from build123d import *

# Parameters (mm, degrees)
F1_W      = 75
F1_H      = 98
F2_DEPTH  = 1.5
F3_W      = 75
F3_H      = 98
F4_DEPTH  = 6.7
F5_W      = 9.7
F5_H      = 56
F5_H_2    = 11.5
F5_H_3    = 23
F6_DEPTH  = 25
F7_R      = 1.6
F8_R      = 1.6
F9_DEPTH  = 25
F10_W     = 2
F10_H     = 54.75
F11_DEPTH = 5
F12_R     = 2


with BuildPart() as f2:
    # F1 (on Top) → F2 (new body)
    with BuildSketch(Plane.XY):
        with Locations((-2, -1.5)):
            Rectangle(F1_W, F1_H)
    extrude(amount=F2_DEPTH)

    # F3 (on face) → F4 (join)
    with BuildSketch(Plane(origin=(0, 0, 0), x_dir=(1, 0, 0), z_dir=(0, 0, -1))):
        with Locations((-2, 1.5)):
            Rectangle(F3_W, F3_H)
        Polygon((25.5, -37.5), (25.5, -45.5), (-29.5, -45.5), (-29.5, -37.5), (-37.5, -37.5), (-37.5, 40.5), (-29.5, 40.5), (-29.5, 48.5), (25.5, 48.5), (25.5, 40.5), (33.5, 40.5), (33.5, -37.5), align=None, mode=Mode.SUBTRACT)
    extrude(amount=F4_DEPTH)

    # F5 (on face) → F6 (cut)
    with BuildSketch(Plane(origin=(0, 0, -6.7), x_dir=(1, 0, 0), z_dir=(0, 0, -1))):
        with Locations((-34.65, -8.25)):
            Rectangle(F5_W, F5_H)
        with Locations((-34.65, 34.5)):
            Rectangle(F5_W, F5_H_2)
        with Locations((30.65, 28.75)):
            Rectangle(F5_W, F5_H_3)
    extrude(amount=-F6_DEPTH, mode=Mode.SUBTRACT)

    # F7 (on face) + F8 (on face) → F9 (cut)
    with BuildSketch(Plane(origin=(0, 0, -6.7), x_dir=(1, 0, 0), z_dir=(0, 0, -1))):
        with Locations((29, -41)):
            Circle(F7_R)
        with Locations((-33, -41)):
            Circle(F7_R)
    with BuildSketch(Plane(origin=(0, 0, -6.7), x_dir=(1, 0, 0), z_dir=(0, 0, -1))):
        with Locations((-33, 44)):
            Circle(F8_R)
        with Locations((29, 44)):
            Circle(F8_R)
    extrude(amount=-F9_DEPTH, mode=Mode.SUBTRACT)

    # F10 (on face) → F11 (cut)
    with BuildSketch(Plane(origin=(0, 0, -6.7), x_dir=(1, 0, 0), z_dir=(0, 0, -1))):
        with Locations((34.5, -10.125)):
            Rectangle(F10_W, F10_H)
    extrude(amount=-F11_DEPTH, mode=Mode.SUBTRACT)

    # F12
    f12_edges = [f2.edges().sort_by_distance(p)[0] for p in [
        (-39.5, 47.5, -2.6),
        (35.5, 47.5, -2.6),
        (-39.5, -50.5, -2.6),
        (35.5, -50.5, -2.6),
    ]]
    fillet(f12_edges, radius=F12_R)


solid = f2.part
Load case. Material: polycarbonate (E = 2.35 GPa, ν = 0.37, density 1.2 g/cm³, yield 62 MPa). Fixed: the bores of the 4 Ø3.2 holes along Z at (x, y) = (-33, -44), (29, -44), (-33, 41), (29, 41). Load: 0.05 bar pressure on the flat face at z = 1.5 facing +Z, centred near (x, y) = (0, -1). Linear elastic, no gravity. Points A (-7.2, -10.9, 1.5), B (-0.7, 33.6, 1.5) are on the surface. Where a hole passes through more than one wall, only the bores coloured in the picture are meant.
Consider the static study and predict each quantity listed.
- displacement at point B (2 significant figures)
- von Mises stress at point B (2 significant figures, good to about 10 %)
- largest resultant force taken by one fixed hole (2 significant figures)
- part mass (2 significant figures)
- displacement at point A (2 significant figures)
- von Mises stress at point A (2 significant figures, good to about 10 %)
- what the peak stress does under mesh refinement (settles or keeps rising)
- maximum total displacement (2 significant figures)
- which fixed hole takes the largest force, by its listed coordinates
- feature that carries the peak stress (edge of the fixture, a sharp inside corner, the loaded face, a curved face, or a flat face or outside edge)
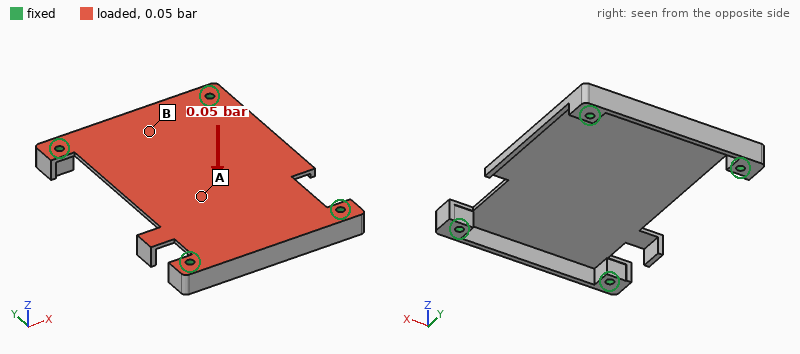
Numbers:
0.36 mm
1.7 MPa
13 N
17 g
1.3 mm
3.8 MPa
keeps rising
1.5 mm
(29, 41)
a sharp inside corner
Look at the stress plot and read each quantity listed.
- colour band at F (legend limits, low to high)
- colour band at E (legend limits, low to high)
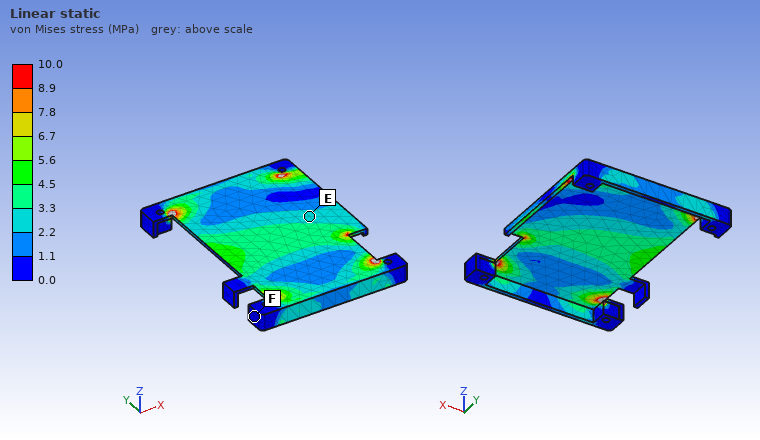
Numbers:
0.0 to 1.1 MPa
2.2 to 3.3 MPa
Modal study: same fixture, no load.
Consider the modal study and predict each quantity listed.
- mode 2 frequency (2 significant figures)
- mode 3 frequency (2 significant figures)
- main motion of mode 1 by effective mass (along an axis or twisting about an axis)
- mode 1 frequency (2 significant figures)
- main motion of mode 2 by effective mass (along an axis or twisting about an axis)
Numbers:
390 Hz
580 Hz
along Z
270 Hz
twisting about Y
